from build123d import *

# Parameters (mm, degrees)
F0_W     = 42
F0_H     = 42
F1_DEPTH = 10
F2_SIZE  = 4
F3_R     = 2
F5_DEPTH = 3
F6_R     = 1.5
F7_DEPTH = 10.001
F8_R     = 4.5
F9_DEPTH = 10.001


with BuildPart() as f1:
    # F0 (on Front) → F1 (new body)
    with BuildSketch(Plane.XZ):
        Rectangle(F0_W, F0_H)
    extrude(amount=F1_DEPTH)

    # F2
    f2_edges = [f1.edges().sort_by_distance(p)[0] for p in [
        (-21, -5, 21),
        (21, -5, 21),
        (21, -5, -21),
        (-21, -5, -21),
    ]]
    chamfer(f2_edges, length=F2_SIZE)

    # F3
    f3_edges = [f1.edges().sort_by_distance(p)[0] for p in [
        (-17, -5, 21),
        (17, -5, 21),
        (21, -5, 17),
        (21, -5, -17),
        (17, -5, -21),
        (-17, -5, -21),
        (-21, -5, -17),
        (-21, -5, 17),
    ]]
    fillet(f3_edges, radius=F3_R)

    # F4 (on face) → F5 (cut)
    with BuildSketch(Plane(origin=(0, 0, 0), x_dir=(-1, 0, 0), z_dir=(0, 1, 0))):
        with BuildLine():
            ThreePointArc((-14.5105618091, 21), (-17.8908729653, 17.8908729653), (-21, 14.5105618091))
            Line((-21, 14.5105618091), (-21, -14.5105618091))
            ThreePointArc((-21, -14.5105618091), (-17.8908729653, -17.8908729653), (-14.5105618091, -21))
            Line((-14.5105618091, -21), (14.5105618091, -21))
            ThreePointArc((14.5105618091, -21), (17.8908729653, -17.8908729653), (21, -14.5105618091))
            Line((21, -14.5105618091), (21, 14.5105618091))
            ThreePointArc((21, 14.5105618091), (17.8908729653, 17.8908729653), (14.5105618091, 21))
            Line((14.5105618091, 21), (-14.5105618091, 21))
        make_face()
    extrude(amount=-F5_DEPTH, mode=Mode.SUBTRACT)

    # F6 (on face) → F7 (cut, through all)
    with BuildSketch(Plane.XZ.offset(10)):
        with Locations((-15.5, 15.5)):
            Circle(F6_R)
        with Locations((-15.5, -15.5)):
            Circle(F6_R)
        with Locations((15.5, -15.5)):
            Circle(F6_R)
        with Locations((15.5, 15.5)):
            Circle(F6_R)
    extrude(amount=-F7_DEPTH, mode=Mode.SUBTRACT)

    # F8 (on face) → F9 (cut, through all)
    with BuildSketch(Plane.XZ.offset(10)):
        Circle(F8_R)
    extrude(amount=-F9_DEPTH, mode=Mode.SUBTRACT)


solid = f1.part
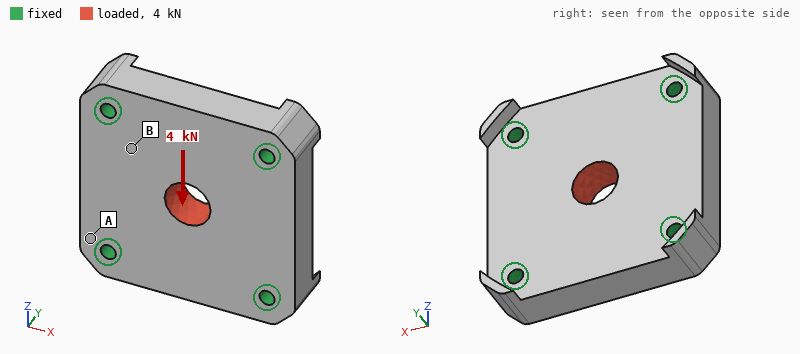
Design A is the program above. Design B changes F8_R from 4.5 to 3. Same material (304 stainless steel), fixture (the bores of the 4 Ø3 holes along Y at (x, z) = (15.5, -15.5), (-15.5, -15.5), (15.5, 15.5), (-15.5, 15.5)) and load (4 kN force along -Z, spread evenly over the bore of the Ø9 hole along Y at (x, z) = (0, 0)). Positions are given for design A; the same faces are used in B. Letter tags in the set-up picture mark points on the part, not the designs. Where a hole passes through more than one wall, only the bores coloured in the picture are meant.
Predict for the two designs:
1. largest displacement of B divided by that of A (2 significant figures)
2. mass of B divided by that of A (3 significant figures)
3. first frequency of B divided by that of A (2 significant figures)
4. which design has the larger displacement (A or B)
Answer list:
1.1
1.02
0.99
B
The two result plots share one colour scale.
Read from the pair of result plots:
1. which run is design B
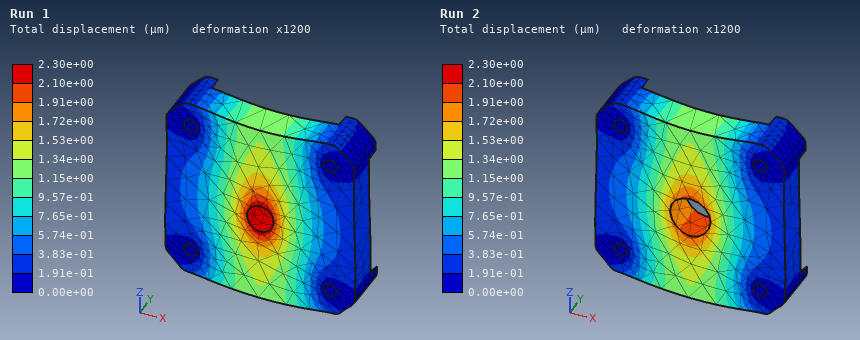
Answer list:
Run 1
